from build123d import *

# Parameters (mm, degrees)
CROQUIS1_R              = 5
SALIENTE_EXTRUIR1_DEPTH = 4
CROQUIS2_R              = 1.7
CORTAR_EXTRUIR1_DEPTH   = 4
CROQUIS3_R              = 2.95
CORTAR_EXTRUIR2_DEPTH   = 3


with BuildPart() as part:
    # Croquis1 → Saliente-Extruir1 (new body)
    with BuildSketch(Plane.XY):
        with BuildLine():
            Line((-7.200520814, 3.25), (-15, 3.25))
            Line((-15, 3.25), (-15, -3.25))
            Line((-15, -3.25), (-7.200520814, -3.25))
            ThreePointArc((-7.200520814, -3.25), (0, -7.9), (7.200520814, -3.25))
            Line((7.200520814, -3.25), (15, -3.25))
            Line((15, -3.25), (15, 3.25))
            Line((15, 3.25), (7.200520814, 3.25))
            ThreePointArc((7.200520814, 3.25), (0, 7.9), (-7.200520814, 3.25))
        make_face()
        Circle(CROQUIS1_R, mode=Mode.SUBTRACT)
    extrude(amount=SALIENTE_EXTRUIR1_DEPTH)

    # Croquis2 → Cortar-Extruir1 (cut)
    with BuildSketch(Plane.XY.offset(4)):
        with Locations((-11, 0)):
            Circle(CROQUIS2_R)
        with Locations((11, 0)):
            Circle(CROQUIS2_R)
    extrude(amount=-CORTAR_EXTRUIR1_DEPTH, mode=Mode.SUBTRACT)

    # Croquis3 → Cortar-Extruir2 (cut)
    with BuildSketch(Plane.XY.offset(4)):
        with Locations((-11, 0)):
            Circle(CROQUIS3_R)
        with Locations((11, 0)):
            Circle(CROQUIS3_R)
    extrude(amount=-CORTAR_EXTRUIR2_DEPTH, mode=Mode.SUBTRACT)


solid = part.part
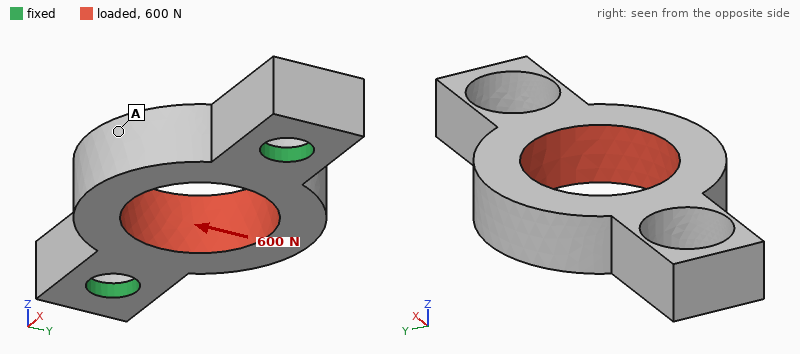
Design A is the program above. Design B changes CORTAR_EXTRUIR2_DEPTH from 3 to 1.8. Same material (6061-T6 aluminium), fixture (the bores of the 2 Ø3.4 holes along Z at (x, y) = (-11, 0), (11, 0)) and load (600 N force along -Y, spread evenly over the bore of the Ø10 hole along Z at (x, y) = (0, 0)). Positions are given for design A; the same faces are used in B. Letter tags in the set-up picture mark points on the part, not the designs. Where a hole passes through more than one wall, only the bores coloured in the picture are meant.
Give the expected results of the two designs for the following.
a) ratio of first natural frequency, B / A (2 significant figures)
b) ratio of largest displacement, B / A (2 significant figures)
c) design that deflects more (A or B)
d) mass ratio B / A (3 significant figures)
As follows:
1.4
0.30
A
1.07
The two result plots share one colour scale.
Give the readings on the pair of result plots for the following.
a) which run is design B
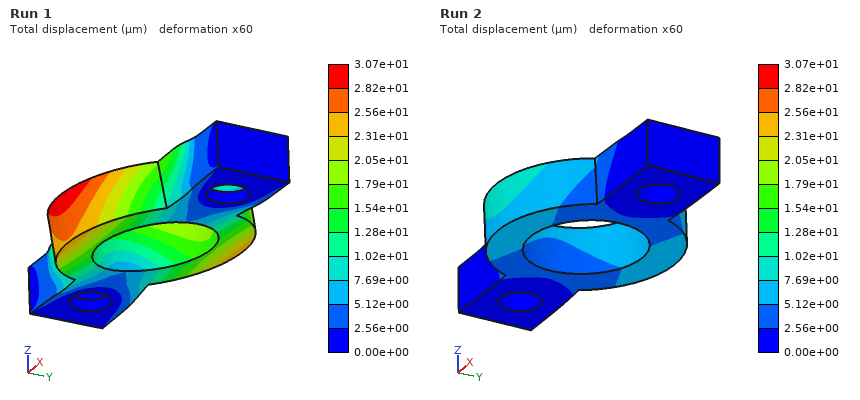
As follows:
Run 2
